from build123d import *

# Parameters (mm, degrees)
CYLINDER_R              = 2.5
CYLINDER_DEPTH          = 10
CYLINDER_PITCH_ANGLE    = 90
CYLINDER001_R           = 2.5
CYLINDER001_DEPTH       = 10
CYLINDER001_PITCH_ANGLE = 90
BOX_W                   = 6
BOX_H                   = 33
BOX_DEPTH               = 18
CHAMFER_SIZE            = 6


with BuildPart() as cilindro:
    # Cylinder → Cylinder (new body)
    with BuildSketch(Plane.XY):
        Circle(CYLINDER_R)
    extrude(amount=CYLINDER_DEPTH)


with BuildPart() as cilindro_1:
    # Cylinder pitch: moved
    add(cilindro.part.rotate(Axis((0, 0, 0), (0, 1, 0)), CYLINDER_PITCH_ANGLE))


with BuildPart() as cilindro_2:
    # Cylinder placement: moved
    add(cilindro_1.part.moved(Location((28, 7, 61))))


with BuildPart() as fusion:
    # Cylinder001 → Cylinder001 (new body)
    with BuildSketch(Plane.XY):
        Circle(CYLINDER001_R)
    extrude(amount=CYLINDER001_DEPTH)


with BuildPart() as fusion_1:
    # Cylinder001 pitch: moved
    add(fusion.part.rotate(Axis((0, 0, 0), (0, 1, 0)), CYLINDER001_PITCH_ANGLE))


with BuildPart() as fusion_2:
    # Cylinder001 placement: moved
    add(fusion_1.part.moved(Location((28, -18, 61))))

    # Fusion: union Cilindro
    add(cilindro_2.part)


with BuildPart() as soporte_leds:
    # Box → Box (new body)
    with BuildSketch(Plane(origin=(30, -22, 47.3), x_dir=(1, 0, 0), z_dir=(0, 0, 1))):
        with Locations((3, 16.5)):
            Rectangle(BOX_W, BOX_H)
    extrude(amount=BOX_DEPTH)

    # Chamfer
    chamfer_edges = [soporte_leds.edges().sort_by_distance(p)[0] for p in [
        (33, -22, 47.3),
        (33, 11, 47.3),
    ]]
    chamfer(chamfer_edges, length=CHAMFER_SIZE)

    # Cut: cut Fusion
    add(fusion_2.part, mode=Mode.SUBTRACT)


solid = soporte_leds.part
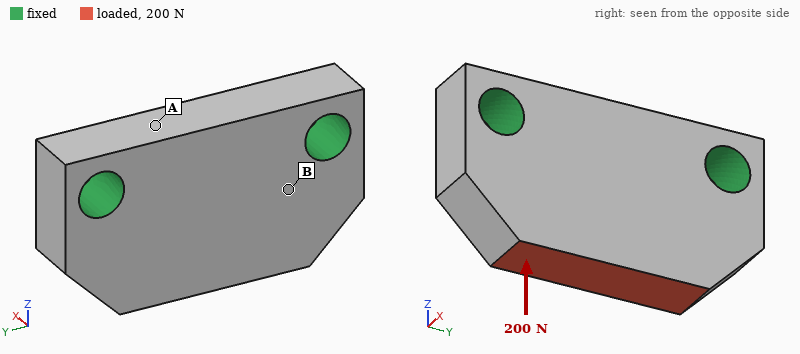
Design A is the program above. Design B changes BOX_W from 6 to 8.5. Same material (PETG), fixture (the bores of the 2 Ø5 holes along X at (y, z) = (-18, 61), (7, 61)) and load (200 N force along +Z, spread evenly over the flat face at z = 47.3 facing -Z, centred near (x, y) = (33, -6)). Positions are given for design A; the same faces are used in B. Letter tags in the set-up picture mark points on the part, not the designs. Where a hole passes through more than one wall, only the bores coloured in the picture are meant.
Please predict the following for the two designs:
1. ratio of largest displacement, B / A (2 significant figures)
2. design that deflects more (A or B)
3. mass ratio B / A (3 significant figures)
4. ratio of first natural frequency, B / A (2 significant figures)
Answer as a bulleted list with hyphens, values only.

- 0.71
- A
- 1.42
- 1.2
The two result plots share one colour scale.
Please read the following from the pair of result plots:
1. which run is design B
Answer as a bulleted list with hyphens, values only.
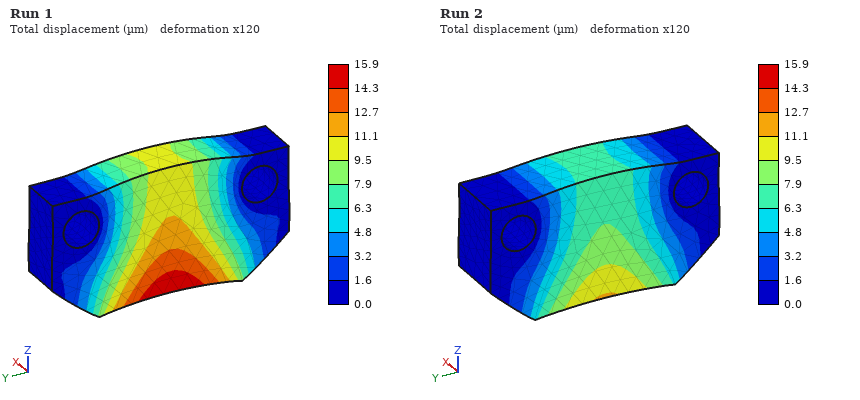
- Run 2
